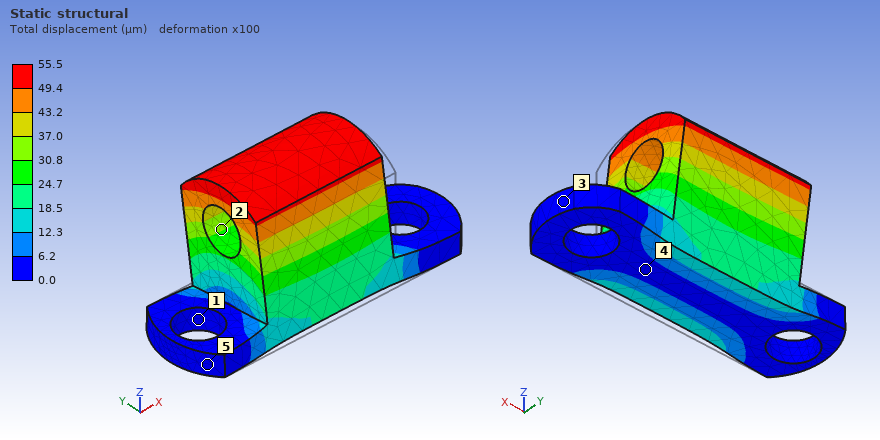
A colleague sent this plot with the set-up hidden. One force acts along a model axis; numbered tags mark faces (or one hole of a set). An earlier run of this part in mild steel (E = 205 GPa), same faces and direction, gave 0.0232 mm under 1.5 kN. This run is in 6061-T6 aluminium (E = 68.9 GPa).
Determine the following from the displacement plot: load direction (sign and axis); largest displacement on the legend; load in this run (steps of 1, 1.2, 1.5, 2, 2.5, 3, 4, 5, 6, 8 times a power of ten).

+Y
55.5 µm
1.2 kN
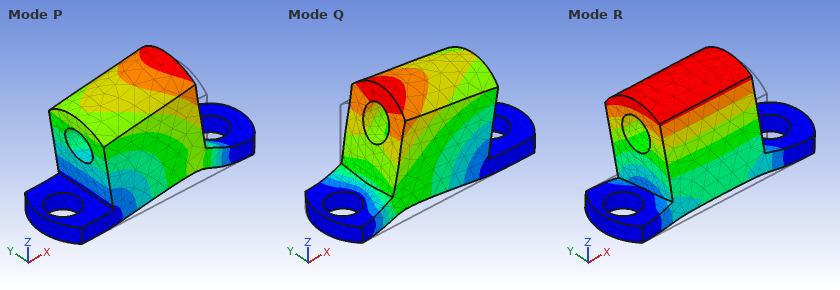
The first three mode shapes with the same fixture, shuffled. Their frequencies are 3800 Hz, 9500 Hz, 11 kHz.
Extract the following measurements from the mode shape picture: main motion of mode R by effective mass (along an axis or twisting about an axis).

along Y
